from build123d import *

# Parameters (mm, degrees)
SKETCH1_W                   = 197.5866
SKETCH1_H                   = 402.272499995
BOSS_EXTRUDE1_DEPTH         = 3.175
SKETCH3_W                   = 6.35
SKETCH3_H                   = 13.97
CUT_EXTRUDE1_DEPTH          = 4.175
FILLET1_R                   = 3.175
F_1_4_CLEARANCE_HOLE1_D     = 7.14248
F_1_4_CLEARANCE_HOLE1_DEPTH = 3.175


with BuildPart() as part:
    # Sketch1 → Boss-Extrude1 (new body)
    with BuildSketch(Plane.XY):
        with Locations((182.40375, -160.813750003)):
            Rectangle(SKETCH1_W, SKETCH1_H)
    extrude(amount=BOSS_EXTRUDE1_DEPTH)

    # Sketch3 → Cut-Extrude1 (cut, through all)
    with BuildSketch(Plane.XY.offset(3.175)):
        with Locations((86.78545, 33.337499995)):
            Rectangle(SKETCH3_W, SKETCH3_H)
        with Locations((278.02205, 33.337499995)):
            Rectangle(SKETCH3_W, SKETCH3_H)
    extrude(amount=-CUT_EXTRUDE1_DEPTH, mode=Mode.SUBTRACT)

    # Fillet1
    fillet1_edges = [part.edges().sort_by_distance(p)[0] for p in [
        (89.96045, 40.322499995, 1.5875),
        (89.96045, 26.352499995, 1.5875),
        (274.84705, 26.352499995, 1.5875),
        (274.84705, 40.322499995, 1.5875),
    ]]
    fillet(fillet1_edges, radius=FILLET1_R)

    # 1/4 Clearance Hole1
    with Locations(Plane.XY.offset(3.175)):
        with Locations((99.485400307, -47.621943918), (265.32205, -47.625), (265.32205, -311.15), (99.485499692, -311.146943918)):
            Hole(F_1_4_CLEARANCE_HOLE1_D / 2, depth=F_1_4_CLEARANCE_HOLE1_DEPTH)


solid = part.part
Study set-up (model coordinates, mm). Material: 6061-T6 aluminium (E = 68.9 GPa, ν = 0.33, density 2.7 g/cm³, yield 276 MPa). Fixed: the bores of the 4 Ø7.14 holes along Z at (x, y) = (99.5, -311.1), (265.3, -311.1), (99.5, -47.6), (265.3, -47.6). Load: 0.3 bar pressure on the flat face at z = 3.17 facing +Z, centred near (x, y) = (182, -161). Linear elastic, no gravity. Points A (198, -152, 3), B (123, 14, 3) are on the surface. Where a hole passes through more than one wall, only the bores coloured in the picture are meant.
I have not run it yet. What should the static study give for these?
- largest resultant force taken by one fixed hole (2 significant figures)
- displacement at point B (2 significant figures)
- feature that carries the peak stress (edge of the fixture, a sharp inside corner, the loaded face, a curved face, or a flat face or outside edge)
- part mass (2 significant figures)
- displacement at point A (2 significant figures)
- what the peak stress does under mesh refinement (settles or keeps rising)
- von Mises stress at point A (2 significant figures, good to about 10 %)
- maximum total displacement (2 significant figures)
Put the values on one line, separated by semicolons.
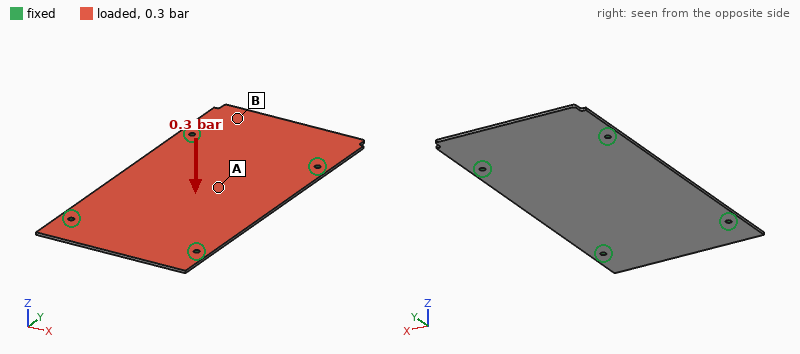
650 N; 0.74 mm; edge of the fixture; 680 g; 2.5 mm; keeps rising; 42 MPa; 2.7 mm
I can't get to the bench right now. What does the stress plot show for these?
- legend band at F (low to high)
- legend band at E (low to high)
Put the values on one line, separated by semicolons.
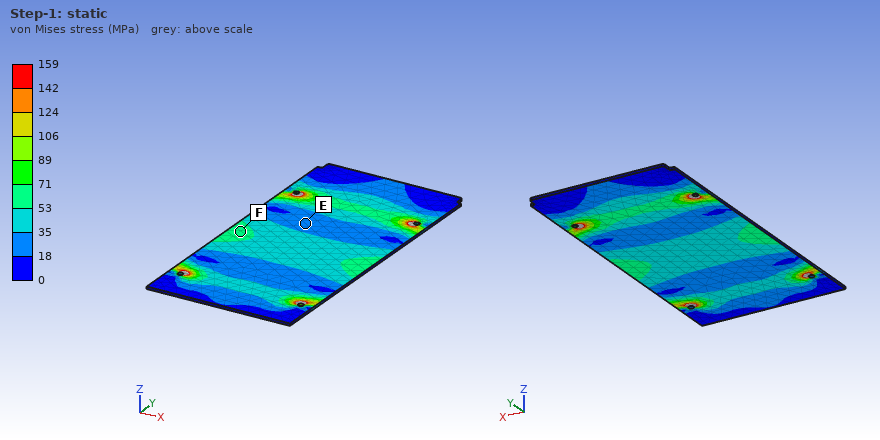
53 to 71 MPa; 18 to 35 MPa
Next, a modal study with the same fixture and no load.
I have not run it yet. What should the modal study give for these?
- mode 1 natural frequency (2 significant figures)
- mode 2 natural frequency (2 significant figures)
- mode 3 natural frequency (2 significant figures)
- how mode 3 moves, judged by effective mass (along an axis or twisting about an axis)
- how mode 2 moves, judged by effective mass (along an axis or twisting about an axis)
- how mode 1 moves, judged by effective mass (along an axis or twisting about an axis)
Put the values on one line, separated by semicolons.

200 Hz; 270 Hz; 320 Hz; twisting about Y; along Z; along Z
